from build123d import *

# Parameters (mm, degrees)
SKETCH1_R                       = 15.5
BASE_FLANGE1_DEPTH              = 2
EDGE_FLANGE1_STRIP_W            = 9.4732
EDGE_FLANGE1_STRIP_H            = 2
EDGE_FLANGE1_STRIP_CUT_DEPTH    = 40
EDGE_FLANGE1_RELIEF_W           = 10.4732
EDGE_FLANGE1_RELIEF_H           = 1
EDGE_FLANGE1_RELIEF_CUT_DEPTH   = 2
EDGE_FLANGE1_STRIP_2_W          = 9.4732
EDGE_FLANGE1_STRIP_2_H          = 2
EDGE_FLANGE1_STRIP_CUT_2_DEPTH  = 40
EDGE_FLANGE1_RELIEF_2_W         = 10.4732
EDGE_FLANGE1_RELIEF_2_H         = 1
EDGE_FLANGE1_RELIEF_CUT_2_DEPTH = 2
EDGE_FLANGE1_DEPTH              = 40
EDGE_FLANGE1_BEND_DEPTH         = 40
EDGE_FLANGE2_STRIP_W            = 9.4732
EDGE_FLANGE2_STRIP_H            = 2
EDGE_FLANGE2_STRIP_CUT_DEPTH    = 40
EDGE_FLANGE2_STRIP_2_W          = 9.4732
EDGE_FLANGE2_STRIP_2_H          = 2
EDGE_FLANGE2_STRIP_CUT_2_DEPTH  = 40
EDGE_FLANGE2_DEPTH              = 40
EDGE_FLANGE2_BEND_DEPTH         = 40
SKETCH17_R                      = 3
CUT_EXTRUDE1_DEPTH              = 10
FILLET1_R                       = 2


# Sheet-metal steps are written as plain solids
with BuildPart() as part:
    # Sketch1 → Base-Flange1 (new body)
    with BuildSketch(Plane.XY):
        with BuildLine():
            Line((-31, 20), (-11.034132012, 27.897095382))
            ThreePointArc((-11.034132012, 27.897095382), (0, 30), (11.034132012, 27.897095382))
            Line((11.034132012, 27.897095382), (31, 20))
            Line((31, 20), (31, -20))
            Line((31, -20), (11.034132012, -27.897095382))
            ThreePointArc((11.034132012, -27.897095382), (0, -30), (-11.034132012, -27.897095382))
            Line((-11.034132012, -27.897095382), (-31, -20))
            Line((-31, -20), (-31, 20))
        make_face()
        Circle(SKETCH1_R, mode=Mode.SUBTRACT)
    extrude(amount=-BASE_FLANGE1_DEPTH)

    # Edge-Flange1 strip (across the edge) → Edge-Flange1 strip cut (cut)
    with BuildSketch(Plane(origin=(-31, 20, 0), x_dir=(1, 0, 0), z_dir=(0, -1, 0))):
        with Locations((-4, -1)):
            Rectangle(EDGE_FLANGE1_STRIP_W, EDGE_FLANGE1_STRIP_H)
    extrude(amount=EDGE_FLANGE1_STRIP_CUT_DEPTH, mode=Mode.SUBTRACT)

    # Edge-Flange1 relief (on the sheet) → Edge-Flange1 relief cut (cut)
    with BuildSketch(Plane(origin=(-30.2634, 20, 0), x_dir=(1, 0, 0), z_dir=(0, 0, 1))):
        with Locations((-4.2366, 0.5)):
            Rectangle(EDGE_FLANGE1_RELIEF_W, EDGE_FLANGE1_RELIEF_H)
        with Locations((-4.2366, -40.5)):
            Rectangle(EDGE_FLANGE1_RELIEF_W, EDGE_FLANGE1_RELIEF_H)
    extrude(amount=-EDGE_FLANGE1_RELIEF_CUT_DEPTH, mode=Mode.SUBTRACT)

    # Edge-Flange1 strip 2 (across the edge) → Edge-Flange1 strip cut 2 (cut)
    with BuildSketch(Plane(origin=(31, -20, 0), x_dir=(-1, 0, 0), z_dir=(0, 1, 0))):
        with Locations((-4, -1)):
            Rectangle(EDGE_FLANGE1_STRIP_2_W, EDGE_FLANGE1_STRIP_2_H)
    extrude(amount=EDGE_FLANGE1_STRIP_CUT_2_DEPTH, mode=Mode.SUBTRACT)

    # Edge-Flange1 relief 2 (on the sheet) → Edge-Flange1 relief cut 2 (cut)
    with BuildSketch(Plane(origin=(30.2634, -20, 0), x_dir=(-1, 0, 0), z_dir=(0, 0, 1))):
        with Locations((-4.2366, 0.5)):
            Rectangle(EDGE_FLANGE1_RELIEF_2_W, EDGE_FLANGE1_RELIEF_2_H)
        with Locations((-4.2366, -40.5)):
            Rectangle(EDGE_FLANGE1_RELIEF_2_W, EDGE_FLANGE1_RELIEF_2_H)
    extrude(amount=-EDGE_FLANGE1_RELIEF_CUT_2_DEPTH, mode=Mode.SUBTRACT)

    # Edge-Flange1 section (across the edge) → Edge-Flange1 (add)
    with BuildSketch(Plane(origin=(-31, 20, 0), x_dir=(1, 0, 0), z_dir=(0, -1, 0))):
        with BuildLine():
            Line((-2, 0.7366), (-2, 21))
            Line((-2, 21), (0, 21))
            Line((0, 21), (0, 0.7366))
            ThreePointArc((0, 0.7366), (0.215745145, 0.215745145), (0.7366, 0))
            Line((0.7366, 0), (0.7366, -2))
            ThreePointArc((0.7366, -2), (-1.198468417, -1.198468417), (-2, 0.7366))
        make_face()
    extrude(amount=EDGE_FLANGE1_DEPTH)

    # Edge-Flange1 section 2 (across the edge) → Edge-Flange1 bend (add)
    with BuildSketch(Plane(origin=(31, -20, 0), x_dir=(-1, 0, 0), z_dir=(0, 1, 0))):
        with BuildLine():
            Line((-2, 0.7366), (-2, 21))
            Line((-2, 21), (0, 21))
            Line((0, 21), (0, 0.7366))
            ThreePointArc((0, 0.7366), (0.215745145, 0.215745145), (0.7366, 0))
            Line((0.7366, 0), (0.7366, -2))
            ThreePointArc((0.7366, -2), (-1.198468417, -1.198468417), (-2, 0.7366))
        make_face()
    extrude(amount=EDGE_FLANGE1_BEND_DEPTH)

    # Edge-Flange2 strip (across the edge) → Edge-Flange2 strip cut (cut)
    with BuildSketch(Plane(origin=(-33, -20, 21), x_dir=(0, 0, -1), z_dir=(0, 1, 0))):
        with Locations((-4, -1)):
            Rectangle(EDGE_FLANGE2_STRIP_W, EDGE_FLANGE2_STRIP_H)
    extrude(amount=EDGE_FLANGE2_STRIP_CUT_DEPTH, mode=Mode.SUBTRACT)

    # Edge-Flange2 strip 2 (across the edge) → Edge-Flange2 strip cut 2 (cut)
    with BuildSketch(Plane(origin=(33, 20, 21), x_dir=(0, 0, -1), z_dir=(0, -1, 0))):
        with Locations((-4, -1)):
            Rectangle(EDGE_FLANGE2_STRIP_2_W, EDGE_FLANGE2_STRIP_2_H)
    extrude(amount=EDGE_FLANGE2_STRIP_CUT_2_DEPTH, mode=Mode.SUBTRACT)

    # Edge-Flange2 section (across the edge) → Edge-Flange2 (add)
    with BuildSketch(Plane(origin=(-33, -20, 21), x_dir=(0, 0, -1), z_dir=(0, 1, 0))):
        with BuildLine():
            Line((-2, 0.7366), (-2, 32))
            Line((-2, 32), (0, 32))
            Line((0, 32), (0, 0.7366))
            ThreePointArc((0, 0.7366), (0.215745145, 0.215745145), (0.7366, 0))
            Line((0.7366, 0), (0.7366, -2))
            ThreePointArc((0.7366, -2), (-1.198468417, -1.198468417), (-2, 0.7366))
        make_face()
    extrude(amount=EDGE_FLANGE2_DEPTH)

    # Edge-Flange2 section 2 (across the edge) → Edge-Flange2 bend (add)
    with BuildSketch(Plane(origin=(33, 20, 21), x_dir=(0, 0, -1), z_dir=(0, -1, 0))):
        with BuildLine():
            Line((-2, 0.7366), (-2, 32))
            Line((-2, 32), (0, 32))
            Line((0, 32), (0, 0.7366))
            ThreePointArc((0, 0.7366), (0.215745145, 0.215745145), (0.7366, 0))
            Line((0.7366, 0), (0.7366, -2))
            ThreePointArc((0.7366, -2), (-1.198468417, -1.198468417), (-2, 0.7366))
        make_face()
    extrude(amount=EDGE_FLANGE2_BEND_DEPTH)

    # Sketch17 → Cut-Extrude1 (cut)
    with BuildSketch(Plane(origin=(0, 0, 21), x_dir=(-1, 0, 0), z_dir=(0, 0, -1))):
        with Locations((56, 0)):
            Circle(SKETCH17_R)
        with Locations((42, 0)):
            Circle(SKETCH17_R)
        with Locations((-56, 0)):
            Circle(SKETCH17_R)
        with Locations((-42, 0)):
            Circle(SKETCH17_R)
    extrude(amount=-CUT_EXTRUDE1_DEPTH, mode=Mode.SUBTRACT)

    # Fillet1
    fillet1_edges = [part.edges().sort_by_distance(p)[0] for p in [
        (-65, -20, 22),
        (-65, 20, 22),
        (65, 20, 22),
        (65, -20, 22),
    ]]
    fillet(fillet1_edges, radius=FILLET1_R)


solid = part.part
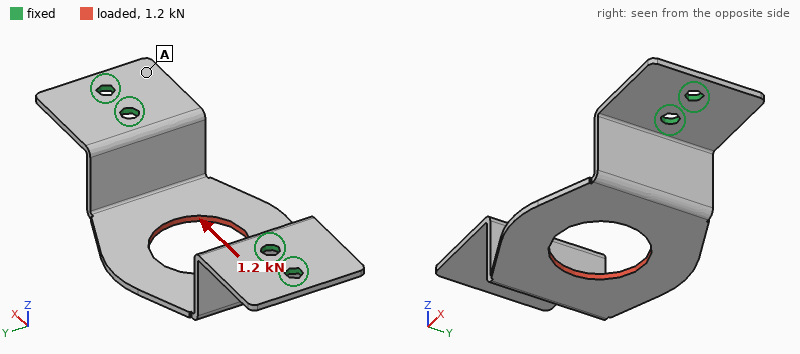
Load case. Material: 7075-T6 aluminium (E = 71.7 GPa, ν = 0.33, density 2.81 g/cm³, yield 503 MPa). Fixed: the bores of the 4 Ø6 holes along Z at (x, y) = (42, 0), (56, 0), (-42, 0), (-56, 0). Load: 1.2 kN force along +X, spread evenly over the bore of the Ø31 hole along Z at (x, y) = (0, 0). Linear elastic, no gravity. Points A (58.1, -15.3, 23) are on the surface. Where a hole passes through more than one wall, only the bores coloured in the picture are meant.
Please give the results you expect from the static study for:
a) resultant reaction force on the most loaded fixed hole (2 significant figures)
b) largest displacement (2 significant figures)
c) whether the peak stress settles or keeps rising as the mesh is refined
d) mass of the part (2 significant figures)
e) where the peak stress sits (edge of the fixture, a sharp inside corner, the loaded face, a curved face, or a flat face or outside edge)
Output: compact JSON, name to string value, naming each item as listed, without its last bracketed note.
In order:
{"resultant reaction force on the most loaded fixed hole": "440 N", "largest displacement": "1.0 mm", "whether the peak stress settles or keeps rising as the mesh is refined": "keeps rising", "mass of the part": "38 g", "where the peak stress sits": "edge of the fixture"}
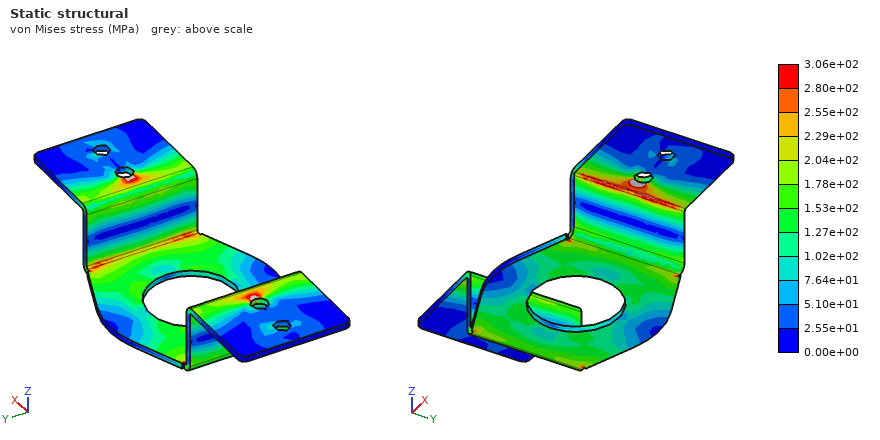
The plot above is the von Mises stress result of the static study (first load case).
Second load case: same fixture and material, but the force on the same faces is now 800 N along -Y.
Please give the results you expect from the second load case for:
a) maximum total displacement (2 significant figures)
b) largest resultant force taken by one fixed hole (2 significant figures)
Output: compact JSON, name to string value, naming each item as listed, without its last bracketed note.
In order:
{"maximum total displacement": "0.73 mm", "largest resultant force taken by one fixed hole": "630 N"}
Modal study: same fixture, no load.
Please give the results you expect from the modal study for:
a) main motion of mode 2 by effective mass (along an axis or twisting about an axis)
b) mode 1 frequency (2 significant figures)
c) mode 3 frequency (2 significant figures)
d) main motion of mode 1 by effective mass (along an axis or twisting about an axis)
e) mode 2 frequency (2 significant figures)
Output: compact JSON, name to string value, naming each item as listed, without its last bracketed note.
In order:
{"main motion of mode 2 by effective mass": "along X", "mode 1 frequency": "1200 Hz", "mode 3 frequency": "1700 Hz", "main motion of mode 1 by effective mass": "along Y", "mode 2 frequency": "1300 Hz"}
